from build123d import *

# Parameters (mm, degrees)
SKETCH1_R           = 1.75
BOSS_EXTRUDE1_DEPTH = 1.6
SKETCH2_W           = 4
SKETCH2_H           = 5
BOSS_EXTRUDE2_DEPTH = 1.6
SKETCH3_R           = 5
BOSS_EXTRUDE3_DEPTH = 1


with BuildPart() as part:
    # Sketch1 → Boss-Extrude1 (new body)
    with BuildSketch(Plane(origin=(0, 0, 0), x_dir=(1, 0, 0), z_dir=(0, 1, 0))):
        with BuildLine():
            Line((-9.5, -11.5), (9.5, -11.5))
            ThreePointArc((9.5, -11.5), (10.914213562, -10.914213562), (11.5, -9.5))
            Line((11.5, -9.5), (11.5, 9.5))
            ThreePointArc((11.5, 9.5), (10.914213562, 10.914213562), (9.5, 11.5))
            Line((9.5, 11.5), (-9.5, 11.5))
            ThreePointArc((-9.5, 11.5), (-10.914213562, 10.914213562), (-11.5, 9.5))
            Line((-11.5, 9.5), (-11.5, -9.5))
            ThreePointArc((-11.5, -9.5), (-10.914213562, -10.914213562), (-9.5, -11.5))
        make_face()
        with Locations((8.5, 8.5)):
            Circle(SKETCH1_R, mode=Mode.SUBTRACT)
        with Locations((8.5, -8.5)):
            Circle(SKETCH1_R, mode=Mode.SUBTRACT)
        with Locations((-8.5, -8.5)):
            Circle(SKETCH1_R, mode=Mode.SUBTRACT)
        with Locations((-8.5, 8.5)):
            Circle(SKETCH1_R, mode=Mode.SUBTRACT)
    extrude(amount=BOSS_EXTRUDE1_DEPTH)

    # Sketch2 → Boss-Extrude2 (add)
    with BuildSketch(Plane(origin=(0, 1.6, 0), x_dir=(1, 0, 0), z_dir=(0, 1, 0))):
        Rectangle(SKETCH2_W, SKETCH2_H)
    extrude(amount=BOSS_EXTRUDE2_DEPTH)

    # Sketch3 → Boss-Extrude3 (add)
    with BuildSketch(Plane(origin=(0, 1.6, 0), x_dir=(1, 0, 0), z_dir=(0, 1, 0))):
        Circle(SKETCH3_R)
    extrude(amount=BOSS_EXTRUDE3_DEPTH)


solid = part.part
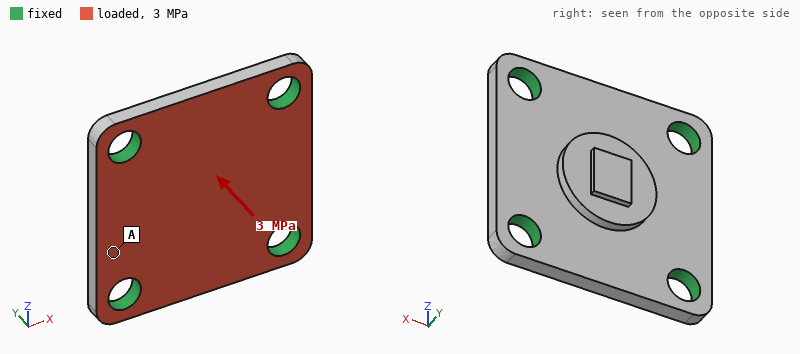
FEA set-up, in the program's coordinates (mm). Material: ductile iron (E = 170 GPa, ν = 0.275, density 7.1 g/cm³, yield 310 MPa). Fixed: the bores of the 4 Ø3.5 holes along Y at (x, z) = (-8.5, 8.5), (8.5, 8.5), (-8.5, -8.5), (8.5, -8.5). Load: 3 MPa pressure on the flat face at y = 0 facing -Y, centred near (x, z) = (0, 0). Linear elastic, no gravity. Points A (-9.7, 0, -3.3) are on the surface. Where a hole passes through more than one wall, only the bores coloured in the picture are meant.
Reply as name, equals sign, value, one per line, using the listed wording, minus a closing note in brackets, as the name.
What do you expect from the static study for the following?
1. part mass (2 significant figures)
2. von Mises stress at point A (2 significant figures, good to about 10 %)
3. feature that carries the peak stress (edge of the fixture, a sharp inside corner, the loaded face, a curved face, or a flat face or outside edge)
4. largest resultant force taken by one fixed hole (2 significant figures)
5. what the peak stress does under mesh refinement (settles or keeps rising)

part mass = 6.2 g
von Mises stress at point A = 31 MPa
feature that carries the peak stress = edge of the fixture
largest resultant force taken by one fixed hole = 370 N
what the peak stress does under mesh refinement = keeps rising
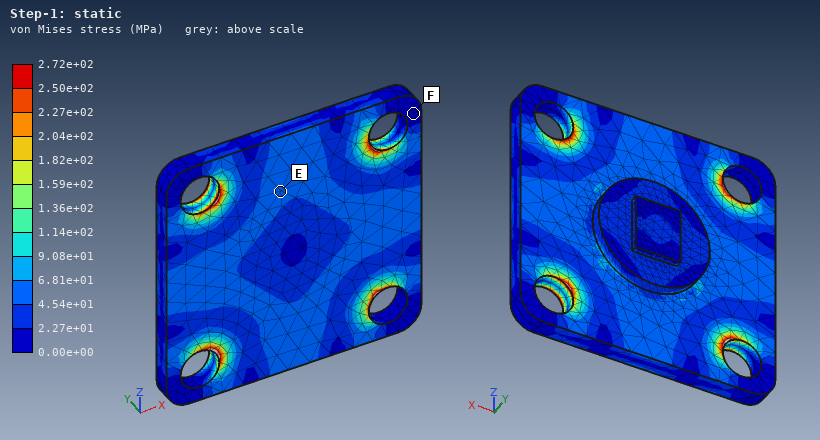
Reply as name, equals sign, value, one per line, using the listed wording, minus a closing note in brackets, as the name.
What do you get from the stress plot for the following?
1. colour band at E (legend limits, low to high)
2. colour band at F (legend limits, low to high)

colour band at E = 4.54e+01 to 6.81e+01 MPa
colour band at F = 0.00e+00 to 2.27e+01 MPa
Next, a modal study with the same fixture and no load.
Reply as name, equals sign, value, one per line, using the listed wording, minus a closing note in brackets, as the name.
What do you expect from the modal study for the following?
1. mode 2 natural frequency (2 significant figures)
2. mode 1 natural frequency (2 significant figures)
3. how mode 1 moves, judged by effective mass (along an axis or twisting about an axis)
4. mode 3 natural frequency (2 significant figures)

mode 2 natural frequency = 38 kHz
mode 1 natural frequency = 25 kHz
how mode 1 moves, judged by effective mass = along Y
mode 3 natural frequency = 38 kHz
